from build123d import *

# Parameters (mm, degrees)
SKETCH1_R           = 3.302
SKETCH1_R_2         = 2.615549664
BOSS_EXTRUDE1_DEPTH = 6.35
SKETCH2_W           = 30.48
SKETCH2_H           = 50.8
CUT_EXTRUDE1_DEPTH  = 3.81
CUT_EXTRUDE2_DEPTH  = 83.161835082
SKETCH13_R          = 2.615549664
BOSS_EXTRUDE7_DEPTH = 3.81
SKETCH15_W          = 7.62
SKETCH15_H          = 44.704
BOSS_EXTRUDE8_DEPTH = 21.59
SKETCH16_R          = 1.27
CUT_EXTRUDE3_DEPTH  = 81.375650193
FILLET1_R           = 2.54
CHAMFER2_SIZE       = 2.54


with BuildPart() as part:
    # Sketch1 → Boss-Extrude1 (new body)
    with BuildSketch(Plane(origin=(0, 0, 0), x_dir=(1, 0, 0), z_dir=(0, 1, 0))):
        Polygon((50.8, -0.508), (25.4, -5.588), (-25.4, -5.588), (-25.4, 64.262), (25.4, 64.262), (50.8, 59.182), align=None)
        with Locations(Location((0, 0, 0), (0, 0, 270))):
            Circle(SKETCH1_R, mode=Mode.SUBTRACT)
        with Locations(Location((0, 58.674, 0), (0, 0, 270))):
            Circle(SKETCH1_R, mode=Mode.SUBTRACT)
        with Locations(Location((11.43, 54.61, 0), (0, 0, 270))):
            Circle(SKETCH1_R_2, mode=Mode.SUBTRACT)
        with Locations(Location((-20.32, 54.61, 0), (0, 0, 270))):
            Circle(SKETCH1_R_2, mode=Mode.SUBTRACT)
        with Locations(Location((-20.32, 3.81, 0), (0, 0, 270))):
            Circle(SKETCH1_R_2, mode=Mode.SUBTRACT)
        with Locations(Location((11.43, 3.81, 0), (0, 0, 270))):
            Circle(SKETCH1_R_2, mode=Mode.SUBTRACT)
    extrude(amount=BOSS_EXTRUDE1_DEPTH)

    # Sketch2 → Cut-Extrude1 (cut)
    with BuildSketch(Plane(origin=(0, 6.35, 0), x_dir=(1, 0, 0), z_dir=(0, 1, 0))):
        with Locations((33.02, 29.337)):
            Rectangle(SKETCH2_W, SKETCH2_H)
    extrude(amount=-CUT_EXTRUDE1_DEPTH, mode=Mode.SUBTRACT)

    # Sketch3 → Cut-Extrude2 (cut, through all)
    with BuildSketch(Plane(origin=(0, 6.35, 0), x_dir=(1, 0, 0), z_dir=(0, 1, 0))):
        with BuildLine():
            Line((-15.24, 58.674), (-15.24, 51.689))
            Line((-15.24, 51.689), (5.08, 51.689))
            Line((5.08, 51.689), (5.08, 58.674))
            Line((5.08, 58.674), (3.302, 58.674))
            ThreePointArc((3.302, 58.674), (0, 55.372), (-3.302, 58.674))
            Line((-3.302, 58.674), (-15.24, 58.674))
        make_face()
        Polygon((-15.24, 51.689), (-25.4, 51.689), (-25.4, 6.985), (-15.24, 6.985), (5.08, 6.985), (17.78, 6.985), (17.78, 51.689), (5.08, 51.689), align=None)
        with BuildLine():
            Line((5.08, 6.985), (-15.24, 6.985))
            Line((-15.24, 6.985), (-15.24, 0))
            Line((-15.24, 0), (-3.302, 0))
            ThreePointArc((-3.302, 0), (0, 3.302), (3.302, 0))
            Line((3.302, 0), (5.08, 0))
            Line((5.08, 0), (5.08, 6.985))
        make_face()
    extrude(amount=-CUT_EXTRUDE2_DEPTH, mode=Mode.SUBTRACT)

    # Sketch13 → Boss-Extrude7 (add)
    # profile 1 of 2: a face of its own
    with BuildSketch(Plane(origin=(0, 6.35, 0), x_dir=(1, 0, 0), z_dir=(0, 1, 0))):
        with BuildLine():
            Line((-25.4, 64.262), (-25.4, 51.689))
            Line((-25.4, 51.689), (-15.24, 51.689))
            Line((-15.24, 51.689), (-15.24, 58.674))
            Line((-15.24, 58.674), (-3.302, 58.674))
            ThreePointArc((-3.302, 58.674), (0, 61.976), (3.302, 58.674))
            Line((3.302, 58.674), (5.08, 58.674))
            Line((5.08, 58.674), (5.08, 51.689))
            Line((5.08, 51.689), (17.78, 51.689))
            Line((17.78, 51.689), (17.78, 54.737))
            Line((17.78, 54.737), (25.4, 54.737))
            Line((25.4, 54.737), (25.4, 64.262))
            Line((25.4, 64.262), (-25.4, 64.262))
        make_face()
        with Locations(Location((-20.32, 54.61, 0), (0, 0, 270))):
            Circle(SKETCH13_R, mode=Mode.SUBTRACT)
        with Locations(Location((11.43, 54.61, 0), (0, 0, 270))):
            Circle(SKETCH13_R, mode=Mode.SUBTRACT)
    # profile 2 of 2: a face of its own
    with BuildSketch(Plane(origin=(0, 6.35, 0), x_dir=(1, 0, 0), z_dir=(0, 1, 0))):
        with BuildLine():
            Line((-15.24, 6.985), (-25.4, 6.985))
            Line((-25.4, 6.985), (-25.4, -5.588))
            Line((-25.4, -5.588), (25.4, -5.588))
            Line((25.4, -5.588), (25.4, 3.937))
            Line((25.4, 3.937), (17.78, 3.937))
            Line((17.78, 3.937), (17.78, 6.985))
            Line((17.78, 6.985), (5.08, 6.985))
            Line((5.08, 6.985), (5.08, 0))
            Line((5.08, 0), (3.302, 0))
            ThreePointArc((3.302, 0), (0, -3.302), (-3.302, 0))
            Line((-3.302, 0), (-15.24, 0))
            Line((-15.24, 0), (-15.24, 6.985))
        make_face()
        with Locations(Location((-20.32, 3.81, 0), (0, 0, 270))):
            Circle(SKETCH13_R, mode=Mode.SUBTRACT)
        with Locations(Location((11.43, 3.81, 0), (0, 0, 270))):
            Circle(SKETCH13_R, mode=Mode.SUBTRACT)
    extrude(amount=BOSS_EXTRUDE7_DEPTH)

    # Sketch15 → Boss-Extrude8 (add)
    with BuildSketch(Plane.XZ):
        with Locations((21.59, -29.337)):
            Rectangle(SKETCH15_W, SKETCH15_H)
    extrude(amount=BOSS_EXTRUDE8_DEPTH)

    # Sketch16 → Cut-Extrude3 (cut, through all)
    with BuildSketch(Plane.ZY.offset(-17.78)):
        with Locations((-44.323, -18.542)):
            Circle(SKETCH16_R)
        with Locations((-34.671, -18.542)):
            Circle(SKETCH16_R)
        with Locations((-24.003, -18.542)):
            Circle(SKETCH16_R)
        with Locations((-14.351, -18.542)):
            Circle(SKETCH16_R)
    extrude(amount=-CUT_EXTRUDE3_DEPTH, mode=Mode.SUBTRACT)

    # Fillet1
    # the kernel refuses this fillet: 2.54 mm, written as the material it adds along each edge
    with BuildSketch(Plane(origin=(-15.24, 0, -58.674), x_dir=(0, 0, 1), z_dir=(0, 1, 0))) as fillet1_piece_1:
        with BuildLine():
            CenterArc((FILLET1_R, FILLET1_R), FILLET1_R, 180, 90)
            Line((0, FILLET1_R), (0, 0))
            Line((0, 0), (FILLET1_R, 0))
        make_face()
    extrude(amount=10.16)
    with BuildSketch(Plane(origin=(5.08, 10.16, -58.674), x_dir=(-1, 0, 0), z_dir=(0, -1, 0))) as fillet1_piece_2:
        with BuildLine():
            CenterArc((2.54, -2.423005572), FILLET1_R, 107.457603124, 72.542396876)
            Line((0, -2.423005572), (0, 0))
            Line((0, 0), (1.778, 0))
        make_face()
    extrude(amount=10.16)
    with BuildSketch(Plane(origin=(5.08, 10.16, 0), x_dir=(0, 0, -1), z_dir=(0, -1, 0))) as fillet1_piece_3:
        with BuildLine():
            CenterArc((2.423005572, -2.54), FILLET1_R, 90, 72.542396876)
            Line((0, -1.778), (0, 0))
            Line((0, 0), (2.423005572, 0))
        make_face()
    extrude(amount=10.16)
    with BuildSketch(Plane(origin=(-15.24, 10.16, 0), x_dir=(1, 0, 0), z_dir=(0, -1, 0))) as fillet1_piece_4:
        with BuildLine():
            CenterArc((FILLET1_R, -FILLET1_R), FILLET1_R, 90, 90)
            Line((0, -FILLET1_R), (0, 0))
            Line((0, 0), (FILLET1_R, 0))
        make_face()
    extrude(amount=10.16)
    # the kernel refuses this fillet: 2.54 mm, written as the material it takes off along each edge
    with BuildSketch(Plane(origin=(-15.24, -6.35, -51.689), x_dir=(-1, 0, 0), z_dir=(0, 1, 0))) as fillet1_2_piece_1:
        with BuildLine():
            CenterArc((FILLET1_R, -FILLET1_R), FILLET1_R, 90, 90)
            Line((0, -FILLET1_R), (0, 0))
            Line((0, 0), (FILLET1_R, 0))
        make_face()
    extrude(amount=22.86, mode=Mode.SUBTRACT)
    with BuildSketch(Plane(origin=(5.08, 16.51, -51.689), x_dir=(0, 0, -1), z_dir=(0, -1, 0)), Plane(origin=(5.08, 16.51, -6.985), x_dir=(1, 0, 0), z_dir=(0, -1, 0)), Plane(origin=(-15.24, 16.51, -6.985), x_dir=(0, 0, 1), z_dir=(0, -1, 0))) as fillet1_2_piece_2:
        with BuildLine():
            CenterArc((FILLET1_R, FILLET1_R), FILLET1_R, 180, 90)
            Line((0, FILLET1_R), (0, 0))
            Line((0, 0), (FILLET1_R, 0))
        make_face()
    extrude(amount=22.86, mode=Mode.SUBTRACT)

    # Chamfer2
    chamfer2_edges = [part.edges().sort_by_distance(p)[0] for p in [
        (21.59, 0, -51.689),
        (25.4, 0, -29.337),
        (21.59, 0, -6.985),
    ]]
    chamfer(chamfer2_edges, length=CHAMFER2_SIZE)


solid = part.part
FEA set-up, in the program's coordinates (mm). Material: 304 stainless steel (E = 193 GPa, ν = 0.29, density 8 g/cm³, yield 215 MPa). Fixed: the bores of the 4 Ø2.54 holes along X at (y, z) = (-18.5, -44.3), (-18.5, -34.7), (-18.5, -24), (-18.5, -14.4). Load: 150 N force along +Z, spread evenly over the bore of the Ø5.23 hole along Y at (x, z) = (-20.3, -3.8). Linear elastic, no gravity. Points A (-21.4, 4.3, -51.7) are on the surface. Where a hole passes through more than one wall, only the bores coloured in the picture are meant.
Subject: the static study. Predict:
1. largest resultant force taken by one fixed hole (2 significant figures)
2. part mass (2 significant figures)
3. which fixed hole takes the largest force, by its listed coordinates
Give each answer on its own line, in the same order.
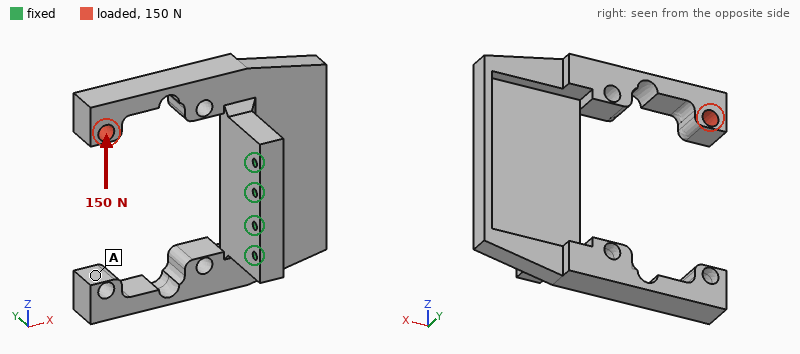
230 N
180 g
(-18.5, -14.4)
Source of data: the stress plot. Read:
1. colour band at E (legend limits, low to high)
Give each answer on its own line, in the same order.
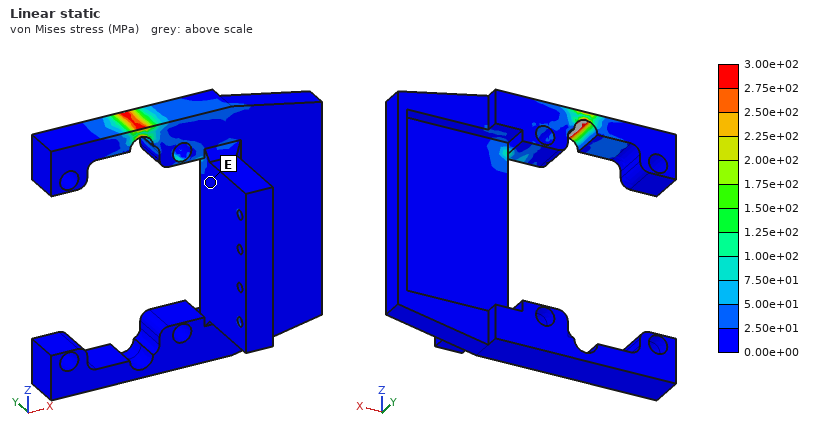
0.00e+00 to 2.50e+01 MPa
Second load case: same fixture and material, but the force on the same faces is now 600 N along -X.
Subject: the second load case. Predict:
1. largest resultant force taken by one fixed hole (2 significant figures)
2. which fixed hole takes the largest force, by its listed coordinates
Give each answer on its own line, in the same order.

520 N
(-18.5, -14.4)
